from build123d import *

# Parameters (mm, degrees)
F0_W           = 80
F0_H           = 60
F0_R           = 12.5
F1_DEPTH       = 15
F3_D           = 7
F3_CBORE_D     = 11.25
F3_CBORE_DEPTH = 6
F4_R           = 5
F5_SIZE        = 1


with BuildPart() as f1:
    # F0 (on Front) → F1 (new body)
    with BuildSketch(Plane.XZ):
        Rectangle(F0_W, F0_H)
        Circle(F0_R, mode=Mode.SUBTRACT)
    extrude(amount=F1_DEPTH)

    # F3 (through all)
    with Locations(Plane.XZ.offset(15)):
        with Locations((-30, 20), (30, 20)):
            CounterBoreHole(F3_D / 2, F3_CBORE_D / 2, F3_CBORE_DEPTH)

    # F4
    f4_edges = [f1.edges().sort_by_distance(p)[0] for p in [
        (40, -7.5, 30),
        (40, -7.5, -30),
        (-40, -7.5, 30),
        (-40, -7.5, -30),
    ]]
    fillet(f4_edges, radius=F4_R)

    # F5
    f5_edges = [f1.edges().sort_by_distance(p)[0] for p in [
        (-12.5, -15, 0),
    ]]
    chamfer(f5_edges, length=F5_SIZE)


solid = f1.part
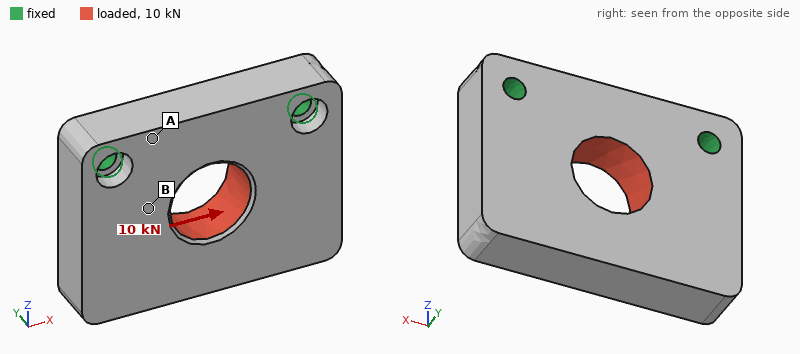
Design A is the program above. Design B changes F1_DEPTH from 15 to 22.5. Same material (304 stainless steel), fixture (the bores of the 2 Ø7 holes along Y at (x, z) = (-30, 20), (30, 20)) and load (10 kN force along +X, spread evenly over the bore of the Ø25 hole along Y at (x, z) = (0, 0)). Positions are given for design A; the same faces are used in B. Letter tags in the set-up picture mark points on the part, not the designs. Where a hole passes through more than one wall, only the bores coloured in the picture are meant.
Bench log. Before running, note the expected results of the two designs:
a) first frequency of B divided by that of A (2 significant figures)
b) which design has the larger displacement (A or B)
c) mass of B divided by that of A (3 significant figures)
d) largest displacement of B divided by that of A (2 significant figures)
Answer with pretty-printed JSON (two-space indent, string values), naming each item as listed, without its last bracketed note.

{
  "first frequency of B divided by that of A": "0.93",
  "which design has the larger displacement": "A",
  "mass of B divided by that of A": "1.49",
  "largest displacement of B divided by that of A": "0.84"
}
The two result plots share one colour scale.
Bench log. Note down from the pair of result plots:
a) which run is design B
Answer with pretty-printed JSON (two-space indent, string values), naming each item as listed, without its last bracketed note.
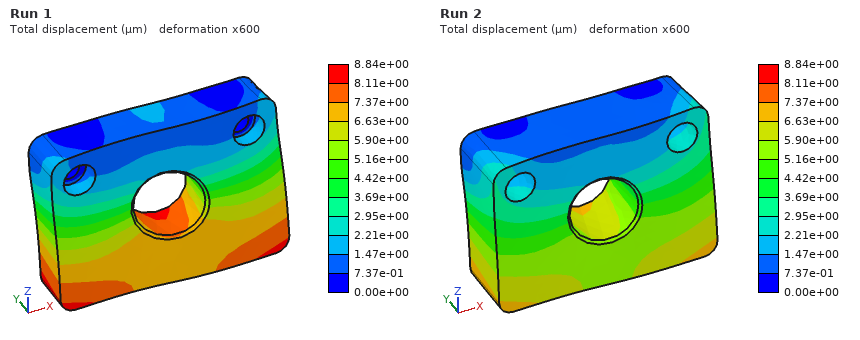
{
  "which run is design B": "Run 2"
}
